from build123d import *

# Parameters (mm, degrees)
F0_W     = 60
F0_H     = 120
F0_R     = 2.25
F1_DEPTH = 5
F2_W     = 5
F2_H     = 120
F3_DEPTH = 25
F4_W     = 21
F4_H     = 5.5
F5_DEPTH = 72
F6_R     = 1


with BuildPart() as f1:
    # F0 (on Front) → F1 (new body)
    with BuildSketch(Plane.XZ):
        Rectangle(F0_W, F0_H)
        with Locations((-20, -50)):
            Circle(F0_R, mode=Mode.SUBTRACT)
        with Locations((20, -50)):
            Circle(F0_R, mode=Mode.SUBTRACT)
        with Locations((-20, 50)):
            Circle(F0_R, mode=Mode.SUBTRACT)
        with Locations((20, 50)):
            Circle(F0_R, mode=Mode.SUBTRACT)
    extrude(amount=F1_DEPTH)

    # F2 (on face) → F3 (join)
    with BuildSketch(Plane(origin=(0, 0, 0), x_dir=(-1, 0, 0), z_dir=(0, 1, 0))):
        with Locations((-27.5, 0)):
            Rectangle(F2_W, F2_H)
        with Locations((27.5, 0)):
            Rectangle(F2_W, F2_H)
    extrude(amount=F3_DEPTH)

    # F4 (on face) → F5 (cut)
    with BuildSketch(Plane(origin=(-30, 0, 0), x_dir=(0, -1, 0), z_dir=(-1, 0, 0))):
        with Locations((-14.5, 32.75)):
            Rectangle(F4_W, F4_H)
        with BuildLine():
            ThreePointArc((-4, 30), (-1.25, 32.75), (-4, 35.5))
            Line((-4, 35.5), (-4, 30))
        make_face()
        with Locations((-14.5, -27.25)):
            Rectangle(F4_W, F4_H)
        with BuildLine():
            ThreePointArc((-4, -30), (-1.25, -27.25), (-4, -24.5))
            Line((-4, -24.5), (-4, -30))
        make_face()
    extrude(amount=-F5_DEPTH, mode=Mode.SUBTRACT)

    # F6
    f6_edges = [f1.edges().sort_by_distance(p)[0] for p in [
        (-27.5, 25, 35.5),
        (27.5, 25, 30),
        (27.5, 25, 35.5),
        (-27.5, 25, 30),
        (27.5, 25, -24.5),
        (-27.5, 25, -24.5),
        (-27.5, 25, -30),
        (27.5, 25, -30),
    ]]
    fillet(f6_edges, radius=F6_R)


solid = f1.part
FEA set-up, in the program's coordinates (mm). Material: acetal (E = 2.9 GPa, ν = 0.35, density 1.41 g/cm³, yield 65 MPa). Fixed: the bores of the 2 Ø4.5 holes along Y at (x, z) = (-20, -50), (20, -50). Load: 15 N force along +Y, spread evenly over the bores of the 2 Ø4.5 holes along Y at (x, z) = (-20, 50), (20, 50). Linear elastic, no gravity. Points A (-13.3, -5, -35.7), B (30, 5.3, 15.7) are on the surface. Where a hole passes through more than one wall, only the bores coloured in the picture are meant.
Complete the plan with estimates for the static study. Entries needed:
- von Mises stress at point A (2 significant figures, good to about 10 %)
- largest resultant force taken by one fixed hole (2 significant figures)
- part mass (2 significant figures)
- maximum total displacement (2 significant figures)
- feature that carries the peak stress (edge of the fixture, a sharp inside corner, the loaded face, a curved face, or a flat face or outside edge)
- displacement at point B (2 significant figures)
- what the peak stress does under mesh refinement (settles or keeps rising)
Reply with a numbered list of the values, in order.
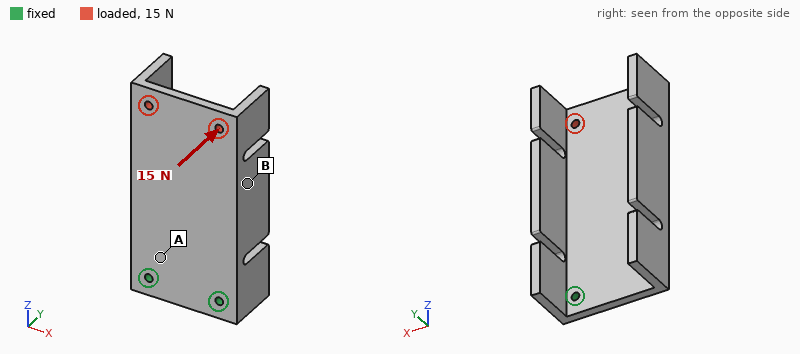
1. 2.4 MPa
2. 12 N
3. 89 g
4. 1.4 mm
5. edge of the fixture
6. 0.66 mm
7. keeps rising
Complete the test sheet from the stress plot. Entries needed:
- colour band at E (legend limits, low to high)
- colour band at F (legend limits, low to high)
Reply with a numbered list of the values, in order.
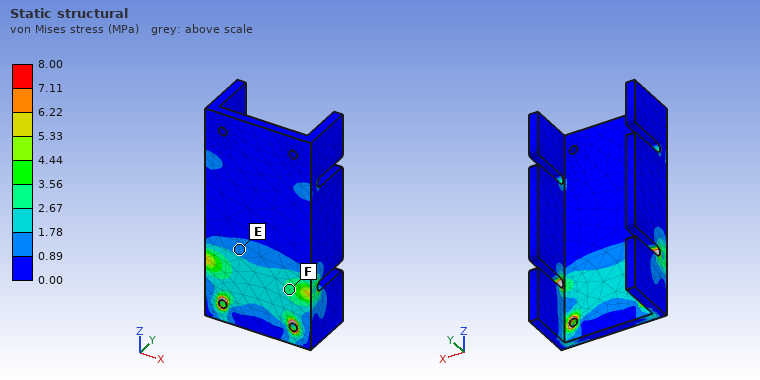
1. 0.89 to 1.78 MPa
2. 2.67 to 3.56 MPa
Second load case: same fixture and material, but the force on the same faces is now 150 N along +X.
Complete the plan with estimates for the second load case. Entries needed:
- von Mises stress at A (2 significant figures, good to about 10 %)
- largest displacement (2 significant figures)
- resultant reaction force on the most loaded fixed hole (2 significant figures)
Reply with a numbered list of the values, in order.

1. 2.5 MPa
2. 0.32 mm
3. 360 N
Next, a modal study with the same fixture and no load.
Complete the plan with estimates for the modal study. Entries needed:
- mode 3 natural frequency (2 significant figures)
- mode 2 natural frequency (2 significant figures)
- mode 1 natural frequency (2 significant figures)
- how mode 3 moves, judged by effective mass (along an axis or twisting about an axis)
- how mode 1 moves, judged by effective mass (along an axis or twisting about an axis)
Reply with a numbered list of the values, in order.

1. 680 Hz
2. 240 Hz
3. 110 Hz
4. along X
5. along Y
